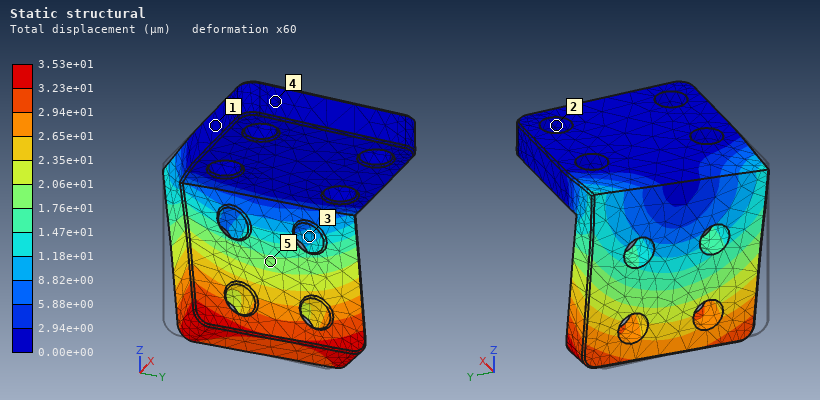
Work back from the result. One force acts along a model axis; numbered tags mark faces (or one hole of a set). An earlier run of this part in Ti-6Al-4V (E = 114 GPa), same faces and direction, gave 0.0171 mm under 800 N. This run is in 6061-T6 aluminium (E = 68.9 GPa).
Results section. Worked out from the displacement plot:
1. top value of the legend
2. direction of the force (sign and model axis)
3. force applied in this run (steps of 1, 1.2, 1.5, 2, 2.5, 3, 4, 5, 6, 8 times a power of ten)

3.53e+01 µm
+Y
1 kN
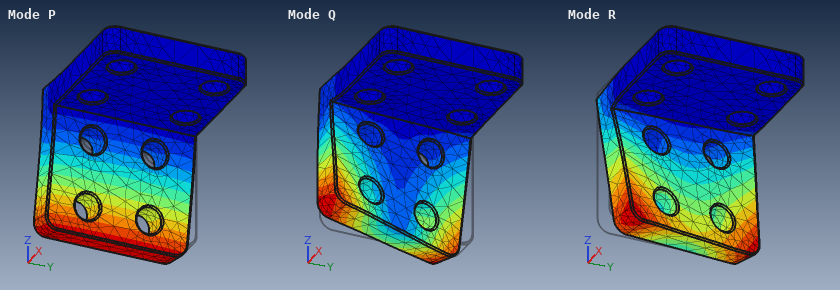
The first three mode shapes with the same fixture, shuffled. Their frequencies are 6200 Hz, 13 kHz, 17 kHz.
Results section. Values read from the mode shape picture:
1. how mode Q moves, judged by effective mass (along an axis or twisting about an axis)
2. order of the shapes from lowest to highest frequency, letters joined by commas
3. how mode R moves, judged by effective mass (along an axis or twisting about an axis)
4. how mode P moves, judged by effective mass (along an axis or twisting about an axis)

along Y
P, R, Q
along Y
along X
